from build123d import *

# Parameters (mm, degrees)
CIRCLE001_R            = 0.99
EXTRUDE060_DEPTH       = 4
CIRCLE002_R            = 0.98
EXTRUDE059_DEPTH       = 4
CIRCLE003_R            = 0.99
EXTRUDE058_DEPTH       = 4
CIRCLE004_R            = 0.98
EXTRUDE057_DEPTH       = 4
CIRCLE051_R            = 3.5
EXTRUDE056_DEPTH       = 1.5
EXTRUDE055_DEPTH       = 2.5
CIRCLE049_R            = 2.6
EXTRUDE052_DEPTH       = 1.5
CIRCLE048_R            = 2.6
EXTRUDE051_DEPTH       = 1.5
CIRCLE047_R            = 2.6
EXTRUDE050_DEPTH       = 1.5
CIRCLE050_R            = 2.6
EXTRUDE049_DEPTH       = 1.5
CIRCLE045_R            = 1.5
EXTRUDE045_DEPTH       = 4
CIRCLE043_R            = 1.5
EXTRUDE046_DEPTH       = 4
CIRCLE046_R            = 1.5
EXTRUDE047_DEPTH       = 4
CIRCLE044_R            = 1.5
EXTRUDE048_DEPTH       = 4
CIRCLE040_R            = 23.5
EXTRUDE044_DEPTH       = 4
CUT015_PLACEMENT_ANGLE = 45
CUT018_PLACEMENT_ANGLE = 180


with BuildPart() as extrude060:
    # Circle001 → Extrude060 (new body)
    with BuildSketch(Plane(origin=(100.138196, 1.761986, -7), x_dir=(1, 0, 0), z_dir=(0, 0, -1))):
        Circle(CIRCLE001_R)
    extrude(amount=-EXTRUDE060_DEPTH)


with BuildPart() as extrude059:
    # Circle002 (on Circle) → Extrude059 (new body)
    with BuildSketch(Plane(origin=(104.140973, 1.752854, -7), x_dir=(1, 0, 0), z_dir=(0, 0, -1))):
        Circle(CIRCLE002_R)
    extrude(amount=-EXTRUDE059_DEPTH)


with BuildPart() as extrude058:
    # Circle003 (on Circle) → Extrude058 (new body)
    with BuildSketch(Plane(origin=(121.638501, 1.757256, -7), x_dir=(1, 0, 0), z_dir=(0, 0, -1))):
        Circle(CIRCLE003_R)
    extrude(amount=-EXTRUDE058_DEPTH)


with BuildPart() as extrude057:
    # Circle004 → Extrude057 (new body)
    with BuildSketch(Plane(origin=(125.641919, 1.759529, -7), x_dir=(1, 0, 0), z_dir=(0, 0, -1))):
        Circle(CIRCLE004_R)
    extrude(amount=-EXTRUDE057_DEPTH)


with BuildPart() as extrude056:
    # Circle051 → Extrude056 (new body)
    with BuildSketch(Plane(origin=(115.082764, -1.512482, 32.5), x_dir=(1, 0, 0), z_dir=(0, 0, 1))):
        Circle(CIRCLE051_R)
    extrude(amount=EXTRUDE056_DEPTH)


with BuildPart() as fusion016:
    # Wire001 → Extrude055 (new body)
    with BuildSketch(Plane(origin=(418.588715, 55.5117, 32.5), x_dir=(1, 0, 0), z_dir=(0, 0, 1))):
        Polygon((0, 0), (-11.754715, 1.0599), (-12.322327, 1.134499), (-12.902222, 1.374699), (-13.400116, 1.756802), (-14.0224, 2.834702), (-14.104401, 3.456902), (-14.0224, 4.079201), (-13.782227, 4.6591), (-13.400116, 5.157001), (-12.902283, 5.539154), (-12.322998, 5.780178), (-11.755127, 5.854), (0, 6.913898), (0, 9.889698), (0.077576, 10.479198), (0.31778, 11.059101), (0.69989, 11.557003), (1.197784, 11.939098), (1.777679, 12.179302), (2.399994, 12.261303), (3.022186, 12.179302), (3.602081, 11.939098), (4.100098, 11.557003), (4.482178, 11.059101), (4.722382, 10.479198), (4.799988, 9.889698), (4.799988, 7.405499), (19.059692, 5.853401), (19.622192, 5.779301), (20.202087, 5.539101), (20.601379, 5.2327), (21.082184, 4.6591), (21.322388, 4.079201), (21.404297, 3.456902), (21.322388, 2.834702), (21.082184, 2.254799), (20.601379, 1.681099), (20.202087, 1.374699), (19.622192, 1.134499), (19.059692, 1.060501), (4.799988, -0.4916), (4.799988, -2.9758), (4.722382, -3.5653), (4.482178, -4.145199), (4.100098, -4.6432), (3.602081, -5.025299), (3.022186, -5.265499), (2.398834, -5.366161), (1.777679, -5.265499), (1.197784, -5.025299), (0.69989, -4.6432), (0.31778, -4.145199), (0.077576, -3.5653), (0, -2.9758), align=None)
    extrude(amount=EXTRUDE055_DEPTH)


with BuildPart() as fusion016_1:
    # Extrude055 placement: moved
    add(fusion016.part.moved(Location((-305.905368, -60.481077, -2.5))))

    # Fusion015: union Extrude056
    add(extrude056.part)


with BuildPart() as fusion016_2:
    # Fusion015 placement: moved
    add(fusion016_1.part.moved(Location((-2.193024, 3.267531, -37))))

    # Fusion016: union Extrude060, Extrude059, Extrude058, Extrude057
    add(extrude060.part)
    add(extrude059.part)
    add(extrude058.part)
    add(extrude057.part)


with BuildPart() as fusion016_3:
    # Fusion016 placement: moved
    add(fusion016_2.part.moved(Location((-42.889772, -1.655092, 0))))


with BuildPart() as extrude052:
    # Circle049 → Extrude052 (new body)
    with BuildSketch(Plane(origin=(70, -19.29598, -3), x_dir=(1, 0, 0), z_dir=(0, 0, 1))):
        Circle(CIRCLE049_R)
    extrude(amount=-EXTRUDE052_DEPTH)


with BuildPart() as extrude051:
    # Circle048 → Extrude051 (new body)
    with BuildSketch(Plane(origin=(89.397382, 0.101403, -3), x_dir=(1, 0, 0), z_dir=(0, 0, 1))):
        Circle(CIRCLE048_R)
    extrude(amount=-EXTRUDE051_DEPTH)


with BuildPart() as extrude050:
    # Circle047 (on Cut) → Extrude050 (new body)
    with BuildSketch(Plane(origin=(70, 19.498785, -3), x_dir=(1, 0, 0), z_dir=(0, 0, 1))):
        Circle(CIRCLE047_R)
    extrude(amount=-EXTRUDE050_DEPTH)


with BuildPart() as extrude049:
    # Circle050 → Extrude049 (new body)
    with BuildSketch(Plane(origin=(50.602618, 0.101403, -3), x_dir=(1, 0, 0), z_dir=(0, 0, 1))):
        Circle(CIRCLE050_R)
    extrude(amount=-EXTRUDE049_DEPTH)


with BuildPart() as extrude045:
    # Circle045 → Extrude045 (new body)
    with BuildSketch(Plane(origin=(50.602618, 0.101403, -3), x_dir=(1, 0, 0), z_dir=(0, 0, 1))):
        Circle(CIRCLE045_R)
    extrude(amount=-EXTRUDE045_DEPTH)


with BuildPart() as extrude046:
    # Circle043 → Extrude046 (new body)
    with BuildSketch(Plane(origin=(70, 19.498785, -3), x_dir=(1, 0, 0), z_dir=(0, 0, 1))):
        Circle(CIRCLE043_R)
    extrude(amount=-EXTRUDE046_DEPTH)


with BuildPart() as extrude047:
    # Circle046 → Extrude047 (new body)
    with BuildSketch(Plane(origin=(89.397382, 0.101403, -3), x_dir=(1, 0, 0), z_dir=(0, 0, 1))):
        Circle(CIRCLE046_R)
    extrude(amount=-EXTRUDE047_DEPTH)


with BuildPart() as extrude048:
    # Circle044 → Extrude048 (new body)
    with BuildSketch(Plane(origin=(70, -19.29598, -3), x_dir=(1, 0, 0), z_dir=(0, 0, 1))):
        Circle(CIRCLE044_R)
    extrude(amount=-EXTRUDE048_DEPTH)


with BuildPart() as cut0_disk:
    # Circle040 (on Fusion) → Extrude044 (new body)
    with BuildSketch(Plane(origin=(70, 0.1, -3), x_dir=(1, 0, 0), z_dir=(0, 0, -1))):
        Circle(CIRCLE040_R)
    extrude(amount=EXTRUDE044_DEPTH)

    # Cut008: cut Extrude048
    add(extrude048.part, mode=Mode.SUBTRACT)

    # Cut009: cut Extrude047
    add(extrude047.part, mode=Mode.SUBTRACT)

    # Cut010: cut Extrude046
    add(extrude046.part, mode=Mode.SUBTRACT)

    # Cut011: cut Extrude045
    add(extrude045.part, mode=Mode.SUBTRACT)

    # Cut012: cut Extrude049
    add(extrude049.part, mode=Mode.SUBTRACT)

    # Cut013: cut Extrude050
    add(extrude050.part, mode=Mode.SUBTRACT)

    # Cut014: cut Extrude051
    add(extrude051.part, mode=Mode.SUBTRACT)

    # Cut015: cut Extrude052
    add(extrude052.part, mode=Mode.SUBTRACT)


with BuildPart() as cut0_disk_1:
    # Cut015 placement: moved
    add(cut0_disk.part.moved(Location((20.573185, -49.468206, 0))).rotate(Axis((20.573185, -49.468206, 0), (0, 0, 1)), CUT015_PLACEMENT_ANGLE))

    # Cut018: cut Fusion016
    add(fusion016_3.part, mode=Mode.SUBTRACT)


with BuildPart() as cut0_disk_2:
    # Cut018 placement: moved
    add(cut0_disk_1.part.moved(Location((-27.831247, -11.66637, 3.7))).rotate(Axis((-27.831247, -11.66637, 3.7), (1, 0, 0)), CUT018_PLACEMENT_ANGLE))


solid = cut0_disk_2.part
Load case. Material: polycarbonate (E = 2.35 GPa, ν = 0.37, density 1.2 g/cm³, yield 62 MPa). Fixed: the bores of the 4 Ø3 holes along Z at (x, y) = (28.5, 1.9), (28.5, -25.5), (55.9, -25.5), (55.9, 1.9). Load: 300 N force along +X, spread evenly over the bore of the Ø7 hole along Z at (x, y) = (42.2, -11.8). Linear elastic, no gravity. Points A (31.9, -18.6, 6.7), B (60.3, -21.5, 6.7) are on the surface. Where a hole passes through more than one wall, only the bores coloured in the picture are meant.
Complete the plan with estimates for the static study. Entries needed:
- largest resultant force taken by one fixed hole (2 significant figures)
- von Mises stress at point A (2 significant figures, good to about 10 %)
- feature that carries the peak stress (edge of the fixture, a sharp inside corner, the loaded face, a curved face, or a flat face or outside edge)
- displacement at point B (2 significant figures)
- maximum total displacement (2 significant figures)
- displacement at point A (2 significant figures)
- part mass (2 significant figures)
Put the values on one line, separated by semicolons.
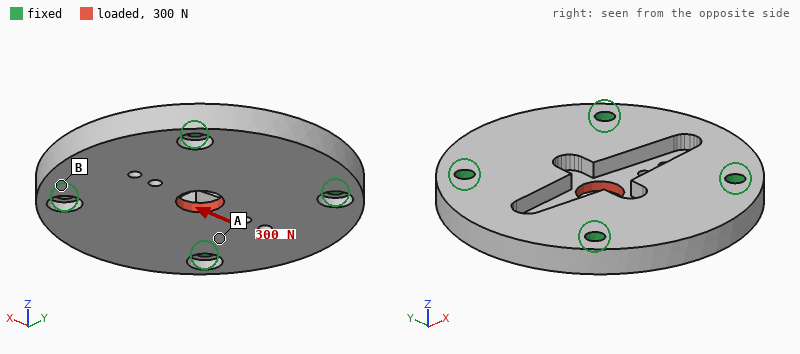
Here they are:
80 N; 2.9 MPa; a sharp inside corner; 12 µm; 46 µm; 14 µm; 7.2 g
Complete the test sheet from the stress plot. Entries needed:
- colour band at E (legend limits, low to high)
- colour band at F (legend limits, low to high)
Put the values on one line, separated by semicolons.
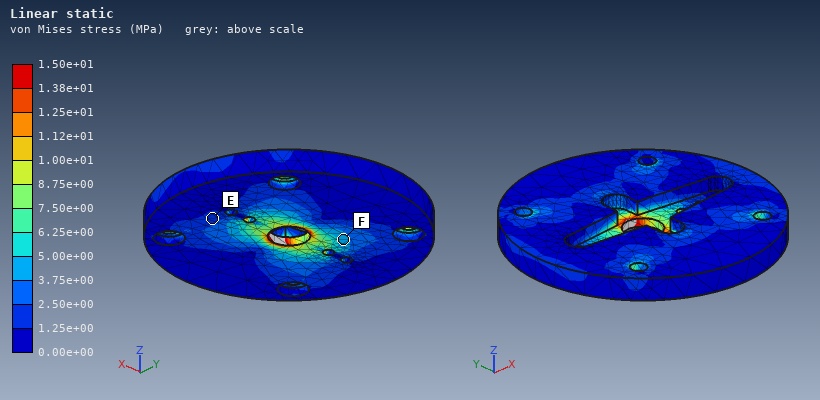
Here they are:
1.25e+00 to 2.50e+00 MPa; 3.75e+00 to 5.00e+00 MPa
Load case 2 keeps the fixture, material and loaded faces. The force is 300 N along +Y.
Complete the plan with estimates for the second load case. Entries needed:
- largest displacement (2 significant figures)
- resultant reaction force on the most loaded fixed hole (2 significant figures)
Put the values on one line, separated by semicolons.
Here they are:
57 µm; 78 N
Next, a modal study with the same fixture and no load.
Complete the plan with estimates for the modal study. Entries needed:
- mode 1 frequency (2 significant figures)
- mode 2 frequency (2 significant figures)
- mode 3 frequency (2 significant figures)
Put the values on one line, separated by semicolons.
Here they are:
4300 Hz; 4600 Hz; 4800 Hz
